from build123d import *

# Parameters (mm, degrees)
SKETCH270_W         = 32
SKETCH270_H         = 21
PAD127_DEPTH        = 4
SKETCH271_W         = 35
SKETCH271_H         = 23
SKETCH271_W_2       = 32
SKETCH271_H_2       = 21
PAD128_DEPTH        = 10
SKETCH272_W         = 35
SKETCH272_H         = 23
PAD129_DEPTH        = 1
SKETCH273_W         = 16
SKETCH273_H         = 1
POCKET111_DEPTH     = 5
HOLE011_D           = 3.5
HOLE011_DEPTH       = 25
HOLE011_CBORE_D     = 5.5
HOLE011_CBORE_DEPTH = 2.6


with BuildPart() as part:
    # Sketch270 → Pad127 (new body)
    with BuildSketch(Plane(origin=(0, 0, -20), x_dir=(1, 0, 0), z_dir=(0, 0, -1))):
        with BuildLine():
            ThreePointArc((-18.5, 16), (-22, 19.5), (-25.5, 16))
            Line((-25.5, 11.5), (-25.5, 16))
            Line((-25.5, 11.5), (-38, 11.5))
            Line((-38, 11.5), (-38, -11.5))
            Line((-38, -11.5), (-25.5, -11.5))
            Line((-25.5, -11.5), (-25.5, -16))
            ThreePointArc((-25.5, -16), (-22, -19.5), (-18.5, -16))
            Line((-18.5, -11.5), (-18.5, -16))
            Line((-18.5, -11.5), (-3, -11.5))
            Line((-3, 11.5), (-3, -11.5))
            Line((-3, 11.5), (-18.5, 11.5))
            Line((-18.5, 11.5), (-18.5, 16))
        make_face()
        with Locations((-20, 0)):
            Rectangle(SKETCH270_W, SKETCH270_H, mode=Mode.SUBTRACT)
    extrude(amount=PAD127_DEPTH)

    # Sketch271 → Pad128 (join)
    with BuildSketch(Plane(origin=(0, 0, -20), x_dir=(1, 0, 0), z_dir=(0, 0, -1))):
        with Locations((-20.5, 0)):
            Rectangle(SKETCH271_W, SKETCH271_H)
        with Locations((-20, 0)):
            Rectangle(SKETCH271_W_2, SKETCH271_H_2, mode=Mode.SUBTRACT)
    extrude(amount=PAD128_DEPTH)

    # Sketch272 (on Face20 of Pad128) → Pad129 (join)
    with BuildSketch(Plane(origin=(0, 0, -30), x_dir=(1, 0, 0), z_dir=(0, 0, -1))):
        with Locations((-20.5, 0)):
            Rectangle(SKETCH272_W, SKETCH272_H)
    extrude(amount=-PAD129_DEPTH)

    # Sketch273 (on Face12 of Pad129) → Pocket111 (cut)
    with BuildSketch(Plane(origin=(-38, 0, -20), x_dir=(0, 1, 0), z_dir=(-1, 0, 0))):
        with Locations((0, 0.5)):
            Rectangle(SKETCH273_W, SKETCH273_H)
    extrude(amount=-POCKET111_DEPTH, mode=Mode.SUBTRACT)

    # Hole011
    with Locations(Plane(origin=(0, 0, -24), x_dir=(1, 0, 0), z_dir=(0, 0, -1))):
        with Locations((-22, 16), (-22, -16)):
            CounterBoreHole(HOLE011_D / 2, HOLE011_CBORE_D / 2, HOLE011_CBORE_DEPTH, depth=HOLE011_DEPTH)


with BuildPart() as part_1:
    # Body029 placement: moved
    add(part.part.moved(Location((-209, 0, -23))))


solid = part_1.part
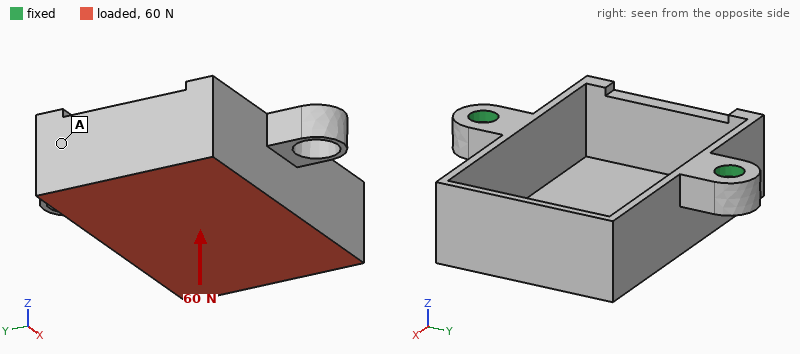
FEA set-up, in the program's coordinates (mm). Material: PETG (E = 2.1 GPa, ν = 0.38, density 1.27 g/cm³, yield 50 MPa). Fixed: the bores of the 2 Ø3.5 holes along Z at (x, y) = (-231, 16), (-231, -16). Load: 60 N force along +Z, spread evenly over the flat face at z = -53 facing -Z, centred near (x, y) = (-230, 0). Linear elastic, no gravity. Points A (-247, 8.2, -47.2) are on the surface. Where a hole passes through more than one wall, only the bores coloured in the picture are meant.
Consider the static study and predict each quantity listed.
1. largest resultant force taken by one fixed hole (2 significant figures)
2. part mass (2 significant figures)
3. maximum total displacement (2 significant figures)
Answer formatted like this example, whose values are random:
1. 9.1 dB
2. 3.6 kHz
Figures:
1. 32 N
2. 2.8 g
3. 0.32 mm
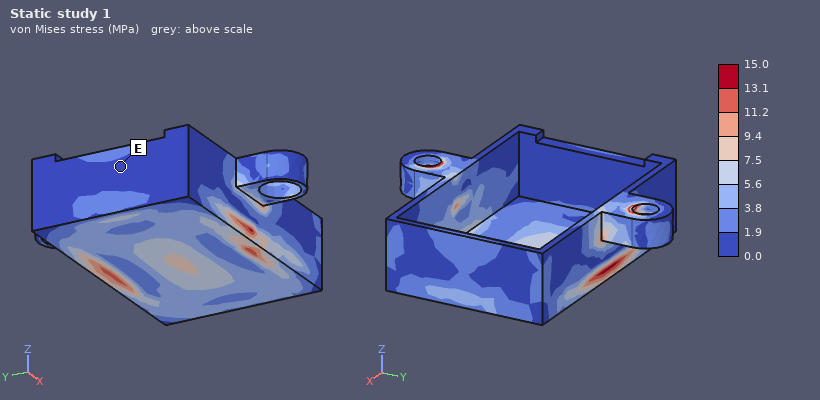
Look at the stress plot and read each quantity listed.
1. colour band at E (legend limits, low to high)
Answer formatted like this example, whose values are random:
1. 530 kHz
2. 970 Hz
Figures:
1. 0.0 to 1.9 MPa
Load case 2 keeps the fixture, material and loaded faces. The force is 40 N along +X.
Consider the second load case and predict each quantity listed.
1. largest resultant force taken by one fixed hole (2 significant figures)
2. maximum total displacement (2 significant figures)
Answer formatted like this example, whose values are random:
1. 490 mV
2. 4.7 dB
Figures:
1. 20 N
2. 0.58 mm
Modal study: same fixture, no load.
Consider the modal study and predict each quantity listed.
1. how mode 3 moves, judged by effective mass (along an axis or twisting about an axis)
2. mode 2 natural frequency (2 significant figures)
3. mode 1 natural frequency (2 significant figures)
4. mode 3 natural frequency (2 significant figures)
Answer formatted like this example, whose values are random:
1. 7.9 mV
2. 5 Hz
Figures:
1. along Y
2. 1000 Hz
3. 830 Hz
4. 1300 Hz
